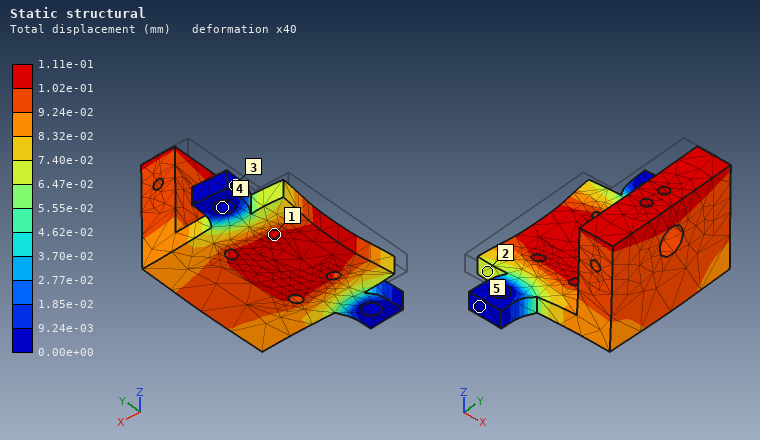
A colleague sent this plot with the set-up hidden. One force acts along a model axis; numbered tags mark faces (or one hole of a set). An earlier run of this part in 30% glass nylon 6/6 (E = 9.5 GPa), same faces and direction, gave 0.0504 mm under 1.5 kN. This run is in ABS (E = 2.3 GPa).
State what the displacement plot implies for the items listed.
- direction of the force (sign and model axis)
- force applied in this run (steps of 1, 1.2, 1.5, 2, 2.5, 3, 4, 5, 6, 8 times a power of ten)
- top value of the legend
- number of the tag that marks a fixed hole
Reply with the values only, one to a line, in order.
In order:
+X
800 N
1.11e-01 mm
4
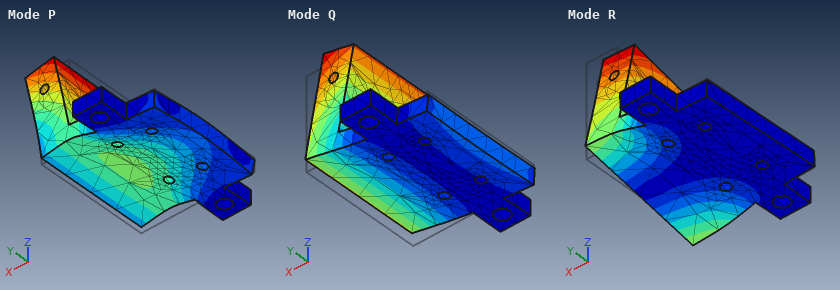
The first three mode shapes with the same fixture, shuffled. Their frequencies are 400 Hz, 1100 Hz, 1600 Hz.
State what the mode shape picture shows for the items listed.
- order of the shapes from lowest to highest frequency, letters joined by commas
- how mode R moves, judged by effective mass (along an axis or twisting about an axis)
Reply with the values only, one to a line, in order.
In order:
Q, R, P
along Y
